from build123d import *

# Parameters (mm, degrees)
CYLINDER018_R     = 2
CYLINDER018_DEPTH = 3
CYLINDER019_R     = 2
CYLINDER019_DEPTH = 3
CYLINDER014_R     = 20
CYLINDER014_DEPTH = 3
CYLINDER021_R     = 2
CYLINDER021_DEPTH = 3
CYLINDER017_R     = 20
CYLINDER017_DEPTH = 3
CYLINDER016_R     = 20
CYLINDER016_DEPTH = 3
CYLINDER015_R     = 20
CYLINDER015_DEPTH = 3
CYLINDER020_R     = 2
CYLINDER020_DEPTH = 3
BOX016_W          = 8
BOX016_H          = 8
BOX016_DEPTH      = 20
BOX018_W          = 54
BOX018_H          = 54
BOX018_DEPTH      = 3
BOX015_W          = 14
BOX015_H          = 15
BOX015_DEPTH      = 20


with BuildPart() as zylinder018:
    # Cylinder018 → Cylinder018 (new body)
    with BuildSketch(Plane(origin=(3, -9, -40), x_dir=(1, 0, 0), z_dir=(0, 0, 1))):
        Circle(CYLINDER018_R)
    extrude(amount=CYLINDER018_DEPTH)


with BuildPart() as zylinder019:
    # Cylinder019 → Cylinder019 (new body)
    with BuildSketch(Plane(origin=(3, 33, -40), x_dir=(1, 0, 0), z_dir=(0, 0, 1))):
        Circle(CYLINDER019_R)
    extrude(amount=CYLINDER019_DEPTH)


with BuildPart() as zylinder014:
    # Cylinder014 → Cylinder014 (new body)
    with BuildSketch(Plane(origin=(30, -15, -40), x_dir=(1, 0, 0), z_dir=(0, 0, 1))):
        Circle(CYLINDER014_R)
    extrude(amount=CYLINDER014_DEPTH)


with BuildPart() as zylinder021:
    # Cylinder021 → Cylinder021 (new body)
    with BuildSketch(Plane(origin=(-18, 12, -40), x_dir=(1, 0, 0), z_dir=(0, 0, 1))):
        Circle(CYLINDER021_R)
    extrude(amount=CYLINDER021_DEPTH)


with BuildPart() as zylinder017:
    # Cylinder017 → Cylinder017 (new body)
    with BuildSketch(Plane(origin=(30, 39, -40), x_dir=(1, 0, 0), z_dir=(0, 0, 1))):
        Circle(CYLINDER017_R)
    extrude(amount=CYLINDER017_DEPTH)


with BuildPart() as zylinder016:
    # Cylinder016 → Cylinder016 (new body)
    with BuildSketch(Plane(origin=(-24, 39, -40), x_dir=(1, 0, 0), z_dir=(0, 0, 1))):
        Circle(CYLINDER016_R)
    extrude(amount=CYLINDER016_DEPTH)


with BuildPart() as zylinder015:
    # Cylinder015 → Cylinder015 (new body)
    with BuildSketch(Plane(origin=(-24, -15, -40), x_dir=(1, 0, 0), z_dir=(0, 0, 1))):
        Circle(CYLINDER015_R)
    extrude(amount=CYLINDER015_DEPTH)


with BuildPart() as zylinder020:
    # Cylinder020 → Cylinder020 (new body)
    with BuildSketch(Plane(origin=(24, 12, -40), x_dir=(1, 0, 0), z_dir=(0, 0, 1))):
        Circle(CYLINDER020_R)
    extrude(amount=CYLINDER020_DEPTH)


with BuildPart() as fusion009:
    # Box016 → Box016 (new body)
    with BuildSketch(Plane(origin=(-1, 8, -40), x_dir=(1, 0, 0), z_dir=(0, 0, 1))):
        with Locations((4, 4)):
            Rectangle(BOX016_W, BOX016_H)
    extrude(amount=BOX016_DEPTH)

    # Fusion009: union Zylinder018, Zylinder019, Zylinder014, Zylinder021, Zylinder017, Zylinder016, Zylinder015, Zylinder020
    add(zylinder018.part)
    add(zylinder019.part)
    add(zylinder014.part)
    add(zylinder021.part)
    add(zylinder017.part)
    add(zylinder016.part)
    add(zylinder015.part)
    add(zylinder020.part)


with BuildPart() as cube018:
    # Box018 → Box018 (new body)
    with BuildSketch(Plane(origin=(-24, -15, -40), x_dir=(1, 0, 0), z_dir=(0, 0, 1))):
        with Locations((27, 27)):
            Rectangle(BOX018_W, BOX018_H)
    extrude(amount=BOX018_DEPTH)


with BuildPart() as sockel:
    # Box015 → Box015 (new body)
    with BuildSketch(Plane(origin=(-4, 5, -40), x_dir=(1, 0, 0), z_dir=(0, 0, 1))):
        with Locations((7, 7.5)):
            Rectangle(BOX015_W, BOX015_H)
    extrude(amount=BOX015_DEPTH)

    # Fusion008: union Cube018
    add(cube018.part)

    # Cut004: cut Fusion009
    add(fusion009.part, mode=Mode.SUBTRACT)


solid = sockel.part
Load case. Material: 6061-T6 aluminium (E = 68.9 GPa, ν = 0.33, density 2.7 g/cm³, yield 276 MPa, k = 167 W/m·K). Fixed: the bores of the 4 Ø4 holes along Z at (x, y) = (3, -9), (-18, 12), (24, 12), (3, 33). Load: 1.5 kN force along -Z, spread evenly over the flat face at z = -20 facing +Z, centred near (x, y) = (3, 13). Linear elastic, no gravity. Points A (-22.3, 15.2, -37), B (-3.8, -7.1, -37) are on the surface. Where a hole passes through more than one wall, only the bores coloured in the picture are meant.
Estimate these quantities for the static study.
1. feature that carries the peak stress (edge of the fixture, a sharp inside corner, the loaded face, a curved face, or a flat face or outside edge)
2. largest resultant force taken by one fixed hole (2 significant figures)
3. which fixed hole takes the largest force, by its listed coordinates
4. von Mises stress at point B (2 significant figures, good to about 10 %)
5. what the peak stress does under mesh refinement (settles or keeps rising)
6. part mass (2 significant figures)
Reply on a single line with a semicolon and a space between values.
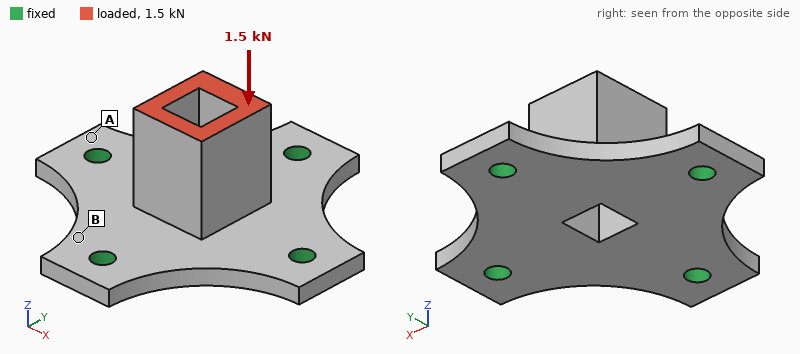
edge of the fixture; 440 N; (3, 33); 28 MPa; keeps rising; 19 g
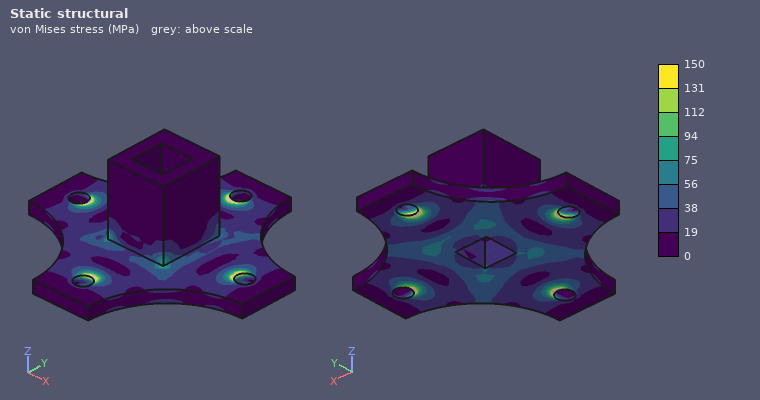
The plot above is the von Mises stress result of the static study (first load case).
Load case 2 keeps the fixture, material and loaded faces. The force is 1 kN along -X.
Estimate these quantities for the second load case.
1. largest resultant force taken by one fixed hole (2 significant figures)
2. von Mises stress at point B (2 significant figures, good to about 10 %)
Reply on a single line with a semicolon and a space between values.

660 N; 18 MPa
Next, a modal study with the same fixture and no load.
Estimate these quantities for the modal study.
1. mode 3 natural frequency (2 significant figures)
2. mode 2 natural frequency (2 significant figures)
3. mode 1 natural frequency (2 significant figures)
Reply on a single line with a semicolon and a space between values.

9900 Hz; 9700 Hz; 9500 Hz
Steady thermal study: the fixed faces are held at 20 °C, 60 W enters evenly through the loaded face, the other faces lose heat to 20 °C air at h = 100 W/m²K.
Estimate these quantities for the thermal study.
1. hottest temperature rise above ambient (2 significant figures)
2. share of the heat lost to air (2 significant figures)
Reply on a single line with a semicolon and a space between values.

64 K; 17 %
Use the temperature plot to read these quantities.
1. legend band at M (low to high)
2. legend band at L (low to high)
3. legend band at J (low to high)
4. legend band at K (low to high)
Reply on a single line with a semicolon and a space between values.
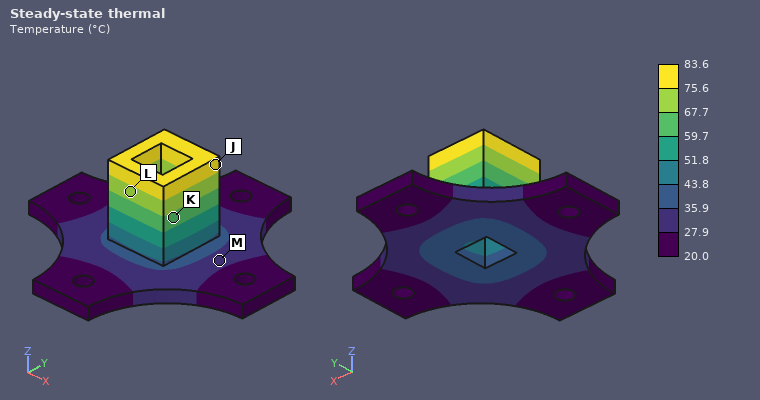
27.9 to 35.9 °C; 67.7 to 75.6 °C; 75.6 to 83.6 °C; 59.7 to 67.7 °C
